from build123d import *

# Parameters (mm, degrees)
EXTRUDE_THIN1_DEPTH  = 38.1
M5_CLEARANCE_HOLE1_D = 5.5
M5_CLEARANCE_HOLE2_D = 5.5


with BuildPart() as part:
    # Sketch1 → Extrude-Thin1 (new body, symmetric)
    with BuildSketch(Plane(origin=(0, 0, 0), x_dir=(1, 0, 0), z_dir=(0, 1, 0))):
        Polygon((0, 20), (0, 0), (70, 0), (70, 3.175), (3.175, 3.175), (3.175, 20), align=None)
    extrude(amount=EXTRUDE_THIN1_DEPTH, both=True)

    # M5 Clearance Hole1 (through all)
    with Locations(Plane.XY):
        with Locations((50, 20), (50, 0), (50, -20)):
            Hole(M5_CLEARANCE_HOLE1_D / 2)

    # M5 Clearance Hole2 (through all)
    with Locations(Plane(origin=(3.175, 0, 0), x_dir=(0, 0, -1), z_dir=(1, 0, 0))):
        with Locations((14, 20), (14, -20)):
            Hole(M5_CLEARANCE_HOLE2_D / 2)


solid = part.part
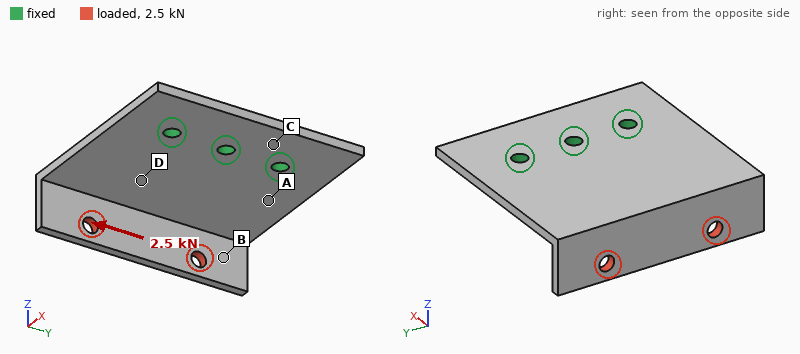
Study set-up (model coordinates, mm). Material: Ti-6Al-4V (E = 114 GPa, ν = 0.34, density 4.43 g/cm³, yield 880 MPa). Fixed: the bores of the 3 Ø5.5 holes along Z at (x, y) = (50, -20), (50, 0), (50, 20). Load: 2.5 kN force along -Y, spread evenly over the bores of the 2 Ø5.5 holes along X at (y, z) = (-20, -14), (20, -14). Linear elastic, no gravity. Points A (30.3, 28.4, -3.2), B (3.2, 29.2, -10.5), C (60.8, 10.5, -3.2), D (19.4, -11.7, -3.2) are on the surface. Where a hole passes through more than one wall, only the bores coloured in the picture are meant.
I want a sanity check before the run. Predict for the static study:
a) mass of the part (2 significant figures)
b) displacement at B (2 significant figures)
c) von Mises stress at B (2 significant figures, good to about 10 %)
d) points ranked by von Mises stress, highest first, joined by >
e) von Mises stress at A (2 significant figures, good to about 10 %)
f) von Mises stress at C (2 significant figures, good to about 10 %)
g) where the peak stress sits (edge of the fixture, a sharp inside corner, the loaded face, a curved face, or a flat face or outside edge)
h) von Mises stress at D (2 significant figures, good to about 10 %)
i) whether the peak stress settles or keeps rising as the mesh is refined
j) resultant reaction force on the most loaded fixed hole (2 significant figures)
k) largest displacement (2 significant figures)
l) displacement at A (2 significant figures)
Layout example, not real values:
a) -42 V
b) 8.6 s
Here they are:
a) 91 g
b) 0.73 mm
c) 82 MPa
d) D > A > B > C
e) 120 MPa
f) 29 MPa
g) edge of the fixture
h) 170 MPa
i) keeps rising
j) 3.0 kN
k) 1.1 mm
l) 0.22 mm
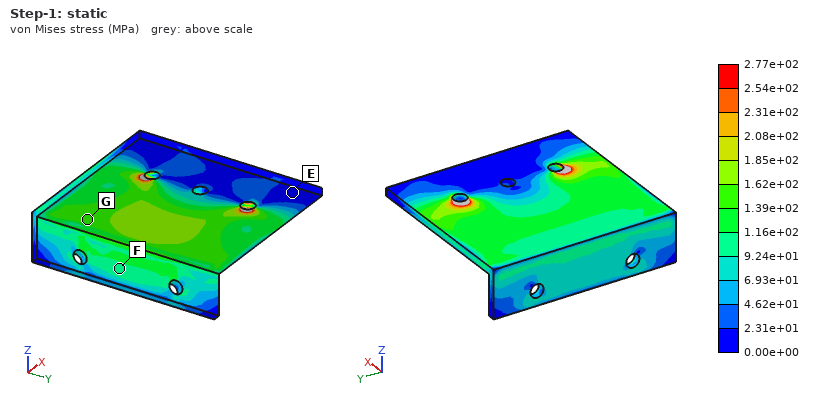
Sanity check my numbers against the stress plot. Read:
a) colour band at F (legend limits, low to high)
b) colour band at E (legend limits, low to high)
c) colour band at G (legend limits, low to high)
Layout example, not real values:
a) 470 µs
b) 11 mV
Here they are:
a) 9.24e+01 to 1.16e+02 MPa
b) 0.00e+00 to 2.31e+01 MPa
c) 1.39e+02 to 1.62e+02 MPa
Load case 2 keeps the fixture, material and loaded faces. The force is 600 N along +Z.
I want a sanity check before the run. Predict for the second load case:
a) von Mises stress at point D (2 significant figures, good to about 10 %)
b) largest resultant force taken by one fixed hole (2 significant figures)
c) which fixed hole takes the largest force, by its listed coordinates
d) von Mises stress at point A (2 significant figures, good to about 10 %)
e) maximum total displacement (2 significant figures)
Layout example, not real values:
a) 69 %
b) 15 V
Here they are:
a) 74 MPa
b) 250 N
c) (50, 0)
d) 120 MPa
e) 1.1 mm
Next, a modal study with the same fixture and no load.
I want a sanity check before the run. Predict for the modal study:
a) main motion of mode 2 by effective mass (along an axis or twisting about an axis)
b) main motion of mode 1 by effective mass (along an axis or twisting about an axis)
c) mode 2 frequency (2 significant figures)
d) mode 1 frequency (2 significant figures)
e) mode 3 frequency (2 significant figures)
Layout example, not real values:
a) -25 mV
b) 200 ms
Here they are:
a) twisting about X
b) along Z
c) 1300 Hz
d) 720 Hz
e) 3600 Hz
